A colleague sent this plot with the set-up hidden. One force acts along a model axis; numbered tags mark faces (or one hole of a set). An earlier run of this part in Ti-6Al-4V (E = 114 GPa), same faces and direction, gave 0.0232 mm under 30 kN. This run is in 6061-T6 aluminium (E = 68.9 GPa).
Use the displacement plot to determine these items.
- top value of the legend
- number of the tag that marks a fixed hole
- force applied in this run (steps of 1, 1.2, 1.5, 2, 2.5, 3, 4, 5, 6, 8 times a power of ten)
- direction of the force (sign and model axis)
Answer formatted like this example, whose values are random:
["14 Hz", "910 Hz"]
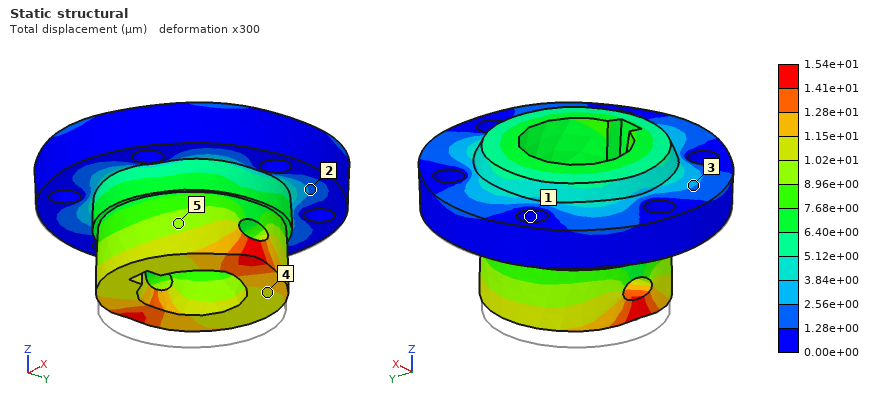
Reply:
["1.54e+01 µm", "1", "12 kN", "+Z"]
